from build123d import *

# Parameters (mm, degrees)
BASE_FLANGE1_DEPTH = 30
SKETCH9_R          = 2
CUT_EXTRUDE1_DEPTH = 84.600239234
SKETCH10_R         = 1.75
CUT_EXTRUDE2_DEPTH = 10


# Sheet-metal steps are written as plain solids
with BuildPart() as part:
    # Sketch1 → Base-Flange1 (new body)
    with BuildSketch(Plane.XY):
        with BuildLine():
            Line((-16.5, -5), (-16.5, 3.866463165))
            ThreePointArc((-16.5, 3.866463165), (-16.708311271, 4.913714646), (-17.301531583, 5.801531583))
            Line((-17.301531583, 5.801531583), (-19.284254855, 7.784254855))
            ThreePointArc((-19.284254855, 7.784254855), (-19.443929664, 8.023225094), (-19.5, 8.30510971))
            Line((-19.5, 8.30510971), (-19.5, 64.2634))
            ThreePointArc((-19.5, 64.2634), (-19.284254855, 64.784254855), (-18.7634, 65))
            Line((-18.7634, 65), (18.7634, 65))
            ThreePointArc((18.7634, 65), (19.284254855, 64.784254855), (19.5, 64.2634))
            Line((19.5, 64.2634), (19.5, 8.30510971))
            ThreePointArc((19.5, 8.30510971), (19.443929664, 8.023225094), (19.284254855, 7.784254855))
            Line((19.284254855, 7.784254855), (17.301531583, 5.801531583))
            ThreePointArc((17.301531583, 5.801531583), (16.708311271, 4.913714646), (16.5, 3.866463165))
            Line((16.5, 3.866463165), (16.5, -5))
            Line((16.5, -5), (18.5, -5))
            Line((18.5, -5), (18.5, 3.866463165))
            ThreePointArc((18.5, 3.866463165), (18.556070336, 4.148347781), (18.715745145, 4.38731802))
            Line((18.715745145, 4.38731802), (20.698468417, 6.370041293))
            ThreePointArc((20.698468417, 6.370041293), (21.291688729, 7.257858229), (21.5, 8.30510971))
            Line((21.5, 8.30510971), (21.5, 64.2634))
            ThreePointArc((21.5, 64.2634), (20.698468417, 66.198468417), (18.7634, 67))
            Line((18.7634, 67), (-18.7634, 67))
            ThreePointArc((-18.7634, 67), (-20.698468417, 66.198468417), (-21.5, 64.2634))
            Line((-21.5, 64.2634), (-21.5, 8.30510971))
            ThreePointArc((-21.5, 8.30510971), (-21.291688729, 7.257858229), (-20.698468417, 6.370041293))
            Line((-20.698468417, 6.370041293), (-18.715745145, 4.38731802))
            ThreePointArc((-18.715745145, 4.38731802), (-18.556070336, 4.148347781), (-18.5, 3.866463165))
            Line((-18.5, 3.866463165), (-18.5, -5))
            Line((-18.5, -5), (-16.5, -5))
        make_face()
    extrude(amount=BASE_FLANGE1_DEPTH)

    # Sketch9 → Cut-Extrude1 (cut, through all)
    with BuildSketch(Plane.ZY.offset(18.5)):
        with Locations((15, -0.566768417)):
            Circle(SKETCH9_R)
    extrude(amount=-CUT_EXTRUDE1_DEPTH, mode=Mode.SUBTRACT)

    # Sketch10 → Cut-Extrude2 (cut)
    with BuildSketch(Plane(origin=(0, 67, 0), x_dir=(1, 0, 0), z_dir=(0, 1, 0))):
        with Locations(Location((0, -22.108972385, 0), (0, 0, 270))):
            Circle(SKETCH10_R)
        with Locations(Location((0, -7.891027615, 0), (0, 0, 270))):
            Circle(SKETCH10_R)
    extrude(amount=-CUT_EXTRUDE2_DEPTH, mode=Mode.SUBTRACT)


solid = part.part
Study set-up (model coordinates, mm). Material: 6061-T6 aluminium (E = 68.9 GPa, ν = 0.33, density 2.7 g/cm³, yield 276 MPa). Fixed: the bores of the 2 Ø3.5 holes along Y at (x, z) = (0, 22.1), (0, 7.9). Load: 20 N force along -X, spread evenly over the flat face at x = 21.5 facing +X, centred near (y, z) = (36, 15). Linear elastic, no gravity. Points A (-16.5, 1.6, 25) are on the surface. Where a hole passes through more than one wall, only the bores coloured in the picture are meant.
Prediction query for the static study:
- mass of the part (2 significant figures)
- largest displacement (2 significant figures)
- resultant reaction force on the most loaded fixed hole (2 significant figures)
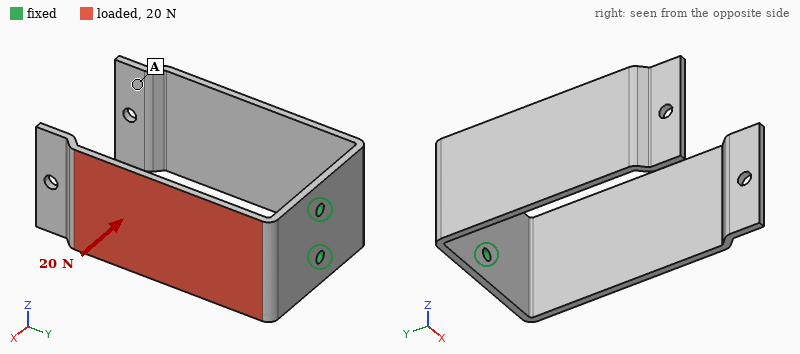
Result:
30 g
0.99 mm
11 N
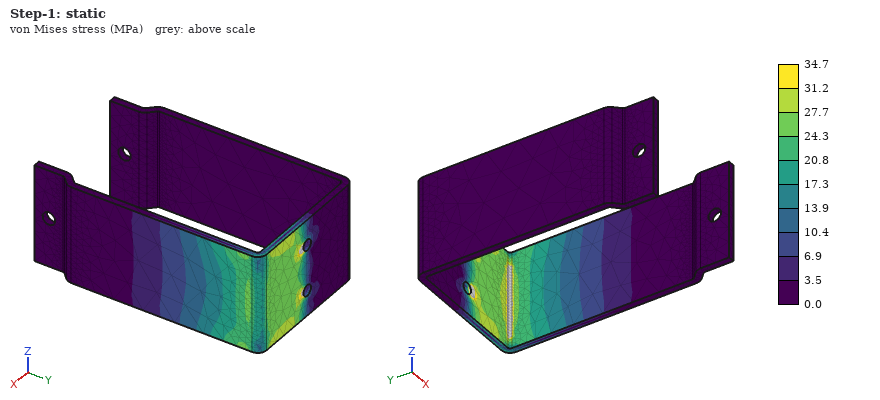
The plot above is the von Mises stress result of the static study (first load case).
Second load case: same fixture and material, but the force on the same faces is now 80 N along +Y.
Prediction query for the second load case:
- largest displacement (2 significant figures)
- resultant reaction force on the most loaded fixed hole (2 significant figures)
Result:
0.93 mm
40 N
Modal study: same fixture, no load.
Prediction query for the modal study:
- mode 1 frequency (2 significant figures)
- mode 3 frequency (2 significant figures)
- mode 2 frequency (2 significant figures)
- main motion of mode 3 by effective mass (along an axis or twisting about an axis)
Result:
230 Hz
460 Hz
230 Hz
twisting about Y
